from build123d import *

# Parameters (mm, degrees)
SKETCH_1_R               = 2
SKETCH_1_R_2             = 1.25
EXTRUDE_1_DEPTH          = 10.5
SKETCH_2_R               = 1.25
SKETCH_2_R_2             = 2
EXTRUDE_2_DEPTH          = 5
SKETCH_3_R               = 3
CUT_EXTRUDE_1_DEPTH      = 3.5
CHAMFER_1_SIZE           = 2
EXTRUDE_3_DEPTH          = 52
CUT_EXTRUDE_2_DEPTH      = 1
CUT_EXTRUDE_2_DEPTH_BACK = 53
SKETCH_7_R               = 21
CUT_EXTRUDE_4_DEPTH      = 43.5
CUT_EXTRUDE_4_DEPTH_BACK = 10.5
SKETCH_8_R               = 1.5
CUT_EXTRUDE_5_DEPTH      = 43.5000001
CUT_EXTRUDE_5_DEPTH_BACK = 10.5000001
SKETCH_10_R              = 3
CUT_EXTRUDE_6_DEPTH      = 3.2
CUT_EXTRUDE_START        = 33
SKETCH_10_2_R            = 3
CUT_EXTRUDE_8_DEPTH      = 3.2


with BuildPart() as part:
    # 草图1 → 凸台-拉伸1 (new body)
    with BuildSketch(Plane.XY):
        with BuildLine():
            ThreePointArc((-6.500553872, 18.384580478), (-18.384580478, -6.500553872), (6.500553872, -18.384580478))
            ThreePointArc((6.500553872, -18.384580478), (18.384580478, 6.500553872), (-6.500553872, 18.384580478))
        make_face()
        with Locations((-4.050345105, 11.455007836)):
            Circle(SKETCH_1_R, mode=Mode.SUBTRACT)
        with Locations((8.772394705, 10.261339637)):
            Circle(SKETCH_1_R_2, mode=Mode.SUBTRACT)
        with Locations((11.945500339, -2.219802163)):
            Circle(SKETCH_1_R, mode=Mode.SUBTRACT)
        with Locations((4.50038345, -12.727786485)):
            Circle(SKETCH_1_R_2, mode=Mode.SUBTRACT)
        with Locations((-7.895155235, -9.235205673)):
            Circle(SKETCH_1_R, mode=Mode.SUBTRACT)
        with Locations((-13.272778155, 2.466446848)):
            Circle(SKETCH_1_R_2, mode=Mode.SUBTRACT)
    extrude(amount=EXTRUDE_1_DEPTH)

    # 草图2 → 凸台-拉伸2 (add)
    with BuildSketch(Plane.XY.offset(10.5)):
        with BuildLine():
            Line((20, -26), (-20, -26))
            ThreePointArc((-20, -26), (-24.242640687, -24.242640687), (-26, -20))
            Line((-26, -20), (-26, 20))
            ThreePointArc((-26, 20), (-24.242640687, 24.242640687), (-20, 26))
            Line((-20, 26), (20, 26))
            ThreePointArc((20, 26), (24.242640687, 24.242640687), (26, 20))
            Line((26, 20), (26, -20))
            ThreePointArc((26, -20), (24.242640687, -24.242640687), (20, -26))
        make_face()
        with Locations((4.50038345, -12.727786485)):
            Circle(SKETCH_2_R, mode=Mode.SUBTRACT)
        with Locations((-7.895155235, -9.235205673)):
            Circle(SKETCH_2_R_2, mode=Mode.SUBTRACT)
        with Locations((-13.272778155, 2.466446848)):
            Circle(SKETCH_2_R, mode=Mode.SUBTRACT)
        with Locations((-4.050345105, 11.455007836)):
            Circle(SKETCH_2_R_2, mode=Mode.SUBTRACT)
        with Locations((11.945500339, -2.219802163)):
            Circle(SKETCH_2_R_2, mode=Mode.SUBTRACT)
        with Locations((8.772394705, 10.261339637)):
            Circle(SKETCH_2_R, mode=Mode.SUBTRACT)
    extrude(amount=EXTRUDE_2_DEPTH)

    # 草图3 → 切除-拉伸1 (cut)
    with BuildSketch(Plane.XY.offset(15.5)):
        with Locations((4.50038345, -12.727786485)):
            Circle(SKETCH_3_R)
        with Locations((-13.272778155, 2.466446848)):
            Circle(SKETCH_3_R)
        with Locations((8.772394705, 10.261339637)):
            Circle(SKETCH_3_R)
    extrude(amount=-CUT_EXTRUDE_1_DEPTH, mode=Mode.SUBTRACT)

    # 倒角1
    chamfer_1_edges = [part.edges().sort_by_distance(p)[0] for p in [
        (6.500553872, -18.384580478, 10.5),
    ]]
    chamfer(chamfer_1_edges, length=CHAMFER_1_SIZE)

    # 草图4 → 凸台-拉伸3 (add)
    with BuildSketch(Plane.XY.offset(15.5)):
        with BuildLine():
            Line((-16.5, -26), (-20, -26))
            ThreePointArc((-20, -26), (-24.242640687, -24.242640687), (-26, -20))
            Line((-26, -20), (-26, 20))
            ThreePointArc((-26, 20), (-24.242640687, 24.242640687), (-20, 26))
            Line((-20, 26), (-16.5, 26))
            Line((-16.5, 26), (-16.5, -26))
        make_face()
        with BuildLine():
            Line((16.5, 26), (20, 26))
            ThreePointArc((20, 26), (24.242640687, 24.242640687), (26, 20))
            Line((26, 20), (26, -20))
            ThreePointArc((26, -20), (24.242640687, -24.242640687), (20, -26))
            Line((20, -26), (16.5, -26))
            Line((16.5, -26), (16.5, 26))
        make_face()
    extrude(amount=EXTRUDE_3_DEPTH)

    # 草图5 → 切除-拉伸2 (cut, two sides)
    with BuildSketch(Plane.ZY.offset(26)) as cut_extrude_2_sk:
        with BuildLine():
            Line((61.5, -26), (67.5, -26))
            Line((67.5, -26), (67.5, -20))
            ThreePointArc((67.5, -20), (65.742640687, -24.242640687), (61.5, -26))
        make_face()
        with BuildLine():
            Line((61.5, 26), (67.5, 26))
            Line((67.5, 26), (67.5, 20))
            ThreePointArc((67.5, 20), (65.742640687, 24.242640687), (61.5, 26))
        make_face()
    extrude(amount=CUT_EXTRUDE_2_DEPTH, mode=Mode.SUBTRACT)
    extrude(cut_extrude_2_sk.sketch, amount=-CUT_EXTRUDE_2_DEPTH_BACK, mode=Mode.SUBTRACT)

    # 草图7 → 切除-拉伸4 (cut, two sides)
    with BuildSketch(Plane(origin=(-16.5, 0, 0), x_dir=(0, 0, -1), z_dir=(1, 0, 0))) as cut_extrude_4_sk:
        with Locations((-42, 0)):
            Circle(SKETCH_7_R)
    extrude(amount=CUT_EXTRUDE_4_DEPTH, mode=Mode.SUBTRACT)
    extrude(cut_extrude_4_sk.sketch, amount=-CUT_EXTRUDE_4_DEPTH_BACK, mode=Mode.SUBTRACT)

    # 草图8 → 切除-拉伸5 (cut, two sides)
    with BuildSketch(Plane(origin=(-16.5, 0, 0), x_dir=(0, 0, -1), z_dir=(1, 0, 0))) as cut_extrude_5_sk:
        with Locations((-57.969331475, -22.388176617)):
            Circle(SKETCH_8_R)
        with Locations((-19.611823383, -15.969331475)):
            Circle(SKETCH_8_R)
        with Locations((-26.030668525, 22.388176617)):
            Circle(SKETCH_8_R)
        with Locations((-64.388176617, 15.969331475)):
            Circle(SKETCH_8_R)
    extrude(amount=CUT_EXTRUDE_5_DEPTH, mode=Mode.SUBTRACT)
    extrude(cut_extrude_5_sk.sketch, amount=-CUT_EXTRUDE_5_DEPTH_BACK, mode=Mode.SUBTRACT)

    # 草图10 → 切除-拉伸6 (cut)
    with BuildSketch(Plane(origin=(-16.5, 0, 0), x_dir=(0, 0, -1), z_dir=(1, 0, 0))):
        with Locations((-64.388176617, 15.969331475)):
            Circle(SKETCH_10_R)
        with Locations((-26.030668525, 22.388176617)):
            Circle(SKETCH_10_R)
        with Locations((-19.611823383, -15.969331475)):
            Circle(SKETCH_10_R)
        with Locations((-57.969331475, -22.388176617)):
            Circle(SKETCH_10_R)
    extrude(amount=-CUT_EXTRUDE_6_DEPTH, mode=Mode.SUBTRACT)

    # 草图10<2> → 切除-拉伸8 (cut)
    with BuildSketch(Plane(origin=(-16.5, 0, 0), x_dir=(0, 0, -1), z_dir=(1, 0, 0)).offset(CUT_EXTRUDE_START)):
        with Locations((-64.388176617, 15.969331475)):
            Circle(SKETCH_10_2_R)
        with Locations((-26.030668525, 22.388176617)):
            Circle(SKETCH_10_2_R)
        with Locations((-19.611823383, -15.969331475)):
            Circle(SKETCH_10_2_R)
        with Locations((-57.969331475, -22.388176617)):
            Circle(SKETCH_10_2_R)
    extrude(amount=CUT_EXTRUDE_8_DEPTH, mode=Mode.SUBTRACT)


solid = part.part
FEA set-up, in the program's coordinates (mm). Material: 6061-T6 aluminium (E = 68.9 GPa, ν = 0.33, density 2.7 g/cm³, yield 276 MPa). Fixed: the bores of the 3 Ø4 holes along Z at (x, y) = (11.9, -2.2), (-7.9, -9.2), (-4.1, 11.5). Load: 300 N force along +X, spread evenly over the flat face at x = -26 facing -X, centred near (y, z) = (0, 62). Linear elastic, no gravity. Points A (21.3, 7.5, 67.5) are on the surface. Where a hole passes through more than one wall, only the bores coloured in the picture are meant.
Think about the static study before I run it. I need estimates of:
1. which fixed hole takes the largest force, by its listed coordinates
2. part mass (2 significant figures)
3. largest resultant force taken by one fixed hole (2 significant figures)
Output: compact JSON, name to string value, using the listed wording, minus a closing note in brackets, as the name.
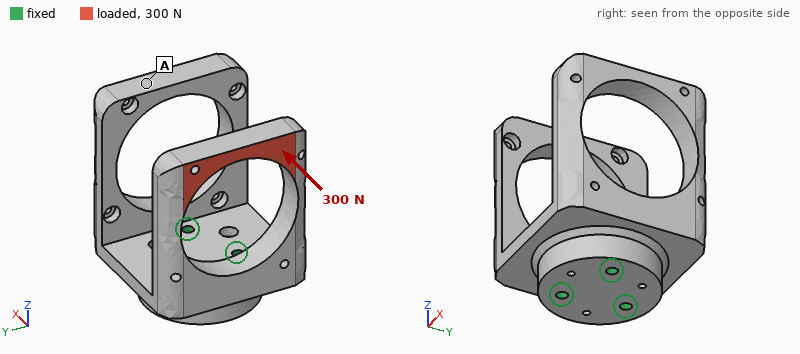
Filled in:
{"which fixed hole takes the largest force, by its listed coordinates": "(-7.9, -9.2)", "part mass": "130 g", "largest resultant force taken by one fixed hole": "250 N"}
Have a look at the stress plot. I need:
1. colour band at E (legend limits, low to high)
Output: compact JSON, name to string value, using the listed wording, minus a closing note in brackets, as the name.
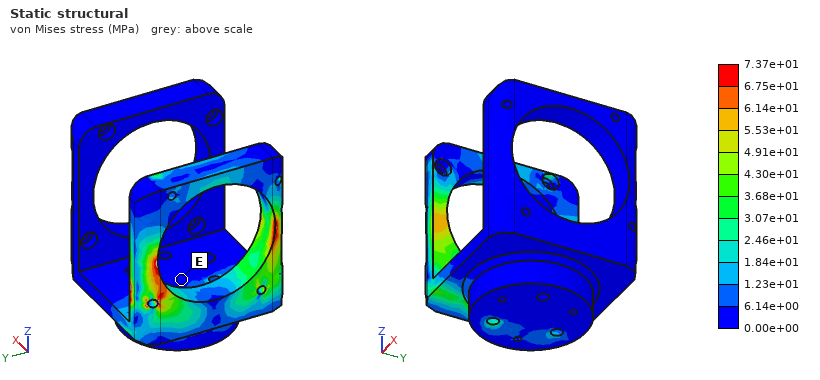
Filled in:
{"colour band at E": "0.00e+00 to 6.14e+00 MPa"}
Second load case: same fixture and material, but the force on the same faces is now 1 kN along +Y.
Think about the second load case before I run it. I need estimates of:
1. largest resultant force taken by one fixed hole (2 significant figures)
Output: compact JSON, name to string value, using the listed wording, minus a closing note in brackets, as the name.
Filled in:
{"largest resultant force taken by one fixed hole": "1.9 kN"}
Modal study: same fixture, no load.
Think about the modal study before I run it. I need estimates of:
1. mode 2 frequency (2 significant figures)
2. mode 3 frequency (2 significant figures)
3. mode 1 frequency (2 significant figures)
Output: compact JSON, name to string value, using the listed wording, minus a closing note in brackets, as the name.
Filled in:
{"mode 2 frequency": "1500 Hz", "mode 3 frequency": "2700 Hz", "mode 1 frequency": "1500 Hz"}
